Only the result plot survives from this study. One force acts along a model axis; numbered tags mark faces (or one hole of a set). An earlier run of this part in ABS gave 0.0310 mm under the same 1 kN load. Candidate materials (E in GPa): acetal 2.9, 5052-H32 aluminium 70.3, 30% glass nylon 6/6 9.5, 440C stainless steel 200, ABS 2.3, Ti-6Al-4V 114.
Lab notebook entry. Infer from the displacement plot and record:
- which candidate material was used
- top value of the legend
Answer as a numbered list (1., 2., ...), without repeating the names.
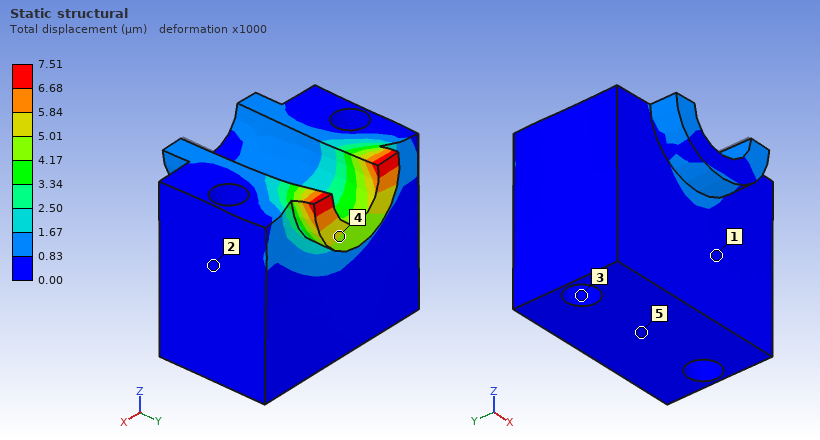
1. 30% glass nylon 6/6
2. 7.51 µm
